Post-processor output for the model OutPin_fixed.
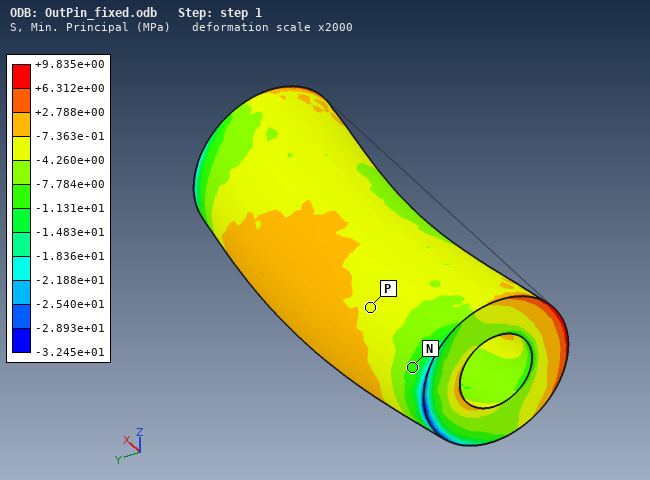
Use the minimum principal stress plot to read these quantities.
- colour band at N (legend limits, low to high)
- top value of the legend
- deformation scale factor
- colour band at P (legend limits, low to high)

-1.131e+01 to -7.784e+00 MPa
+9.835e+00 MPa
2000
-4.260e+00 to -7.363e-01 MPa
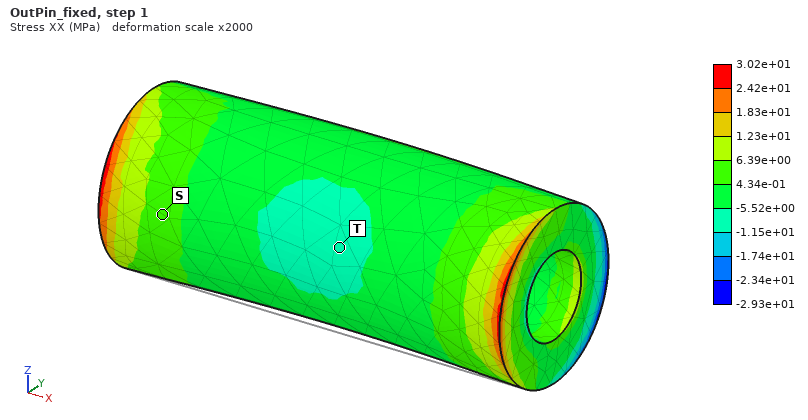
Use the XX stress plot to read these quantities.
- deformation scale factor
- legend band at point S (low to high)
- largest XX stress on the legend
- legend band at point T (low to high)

2000
4.34e-01 to 6.39e+00 MPa
3.02e+01 MPa
-1.15e+01 to -5.52e+00 MPa
